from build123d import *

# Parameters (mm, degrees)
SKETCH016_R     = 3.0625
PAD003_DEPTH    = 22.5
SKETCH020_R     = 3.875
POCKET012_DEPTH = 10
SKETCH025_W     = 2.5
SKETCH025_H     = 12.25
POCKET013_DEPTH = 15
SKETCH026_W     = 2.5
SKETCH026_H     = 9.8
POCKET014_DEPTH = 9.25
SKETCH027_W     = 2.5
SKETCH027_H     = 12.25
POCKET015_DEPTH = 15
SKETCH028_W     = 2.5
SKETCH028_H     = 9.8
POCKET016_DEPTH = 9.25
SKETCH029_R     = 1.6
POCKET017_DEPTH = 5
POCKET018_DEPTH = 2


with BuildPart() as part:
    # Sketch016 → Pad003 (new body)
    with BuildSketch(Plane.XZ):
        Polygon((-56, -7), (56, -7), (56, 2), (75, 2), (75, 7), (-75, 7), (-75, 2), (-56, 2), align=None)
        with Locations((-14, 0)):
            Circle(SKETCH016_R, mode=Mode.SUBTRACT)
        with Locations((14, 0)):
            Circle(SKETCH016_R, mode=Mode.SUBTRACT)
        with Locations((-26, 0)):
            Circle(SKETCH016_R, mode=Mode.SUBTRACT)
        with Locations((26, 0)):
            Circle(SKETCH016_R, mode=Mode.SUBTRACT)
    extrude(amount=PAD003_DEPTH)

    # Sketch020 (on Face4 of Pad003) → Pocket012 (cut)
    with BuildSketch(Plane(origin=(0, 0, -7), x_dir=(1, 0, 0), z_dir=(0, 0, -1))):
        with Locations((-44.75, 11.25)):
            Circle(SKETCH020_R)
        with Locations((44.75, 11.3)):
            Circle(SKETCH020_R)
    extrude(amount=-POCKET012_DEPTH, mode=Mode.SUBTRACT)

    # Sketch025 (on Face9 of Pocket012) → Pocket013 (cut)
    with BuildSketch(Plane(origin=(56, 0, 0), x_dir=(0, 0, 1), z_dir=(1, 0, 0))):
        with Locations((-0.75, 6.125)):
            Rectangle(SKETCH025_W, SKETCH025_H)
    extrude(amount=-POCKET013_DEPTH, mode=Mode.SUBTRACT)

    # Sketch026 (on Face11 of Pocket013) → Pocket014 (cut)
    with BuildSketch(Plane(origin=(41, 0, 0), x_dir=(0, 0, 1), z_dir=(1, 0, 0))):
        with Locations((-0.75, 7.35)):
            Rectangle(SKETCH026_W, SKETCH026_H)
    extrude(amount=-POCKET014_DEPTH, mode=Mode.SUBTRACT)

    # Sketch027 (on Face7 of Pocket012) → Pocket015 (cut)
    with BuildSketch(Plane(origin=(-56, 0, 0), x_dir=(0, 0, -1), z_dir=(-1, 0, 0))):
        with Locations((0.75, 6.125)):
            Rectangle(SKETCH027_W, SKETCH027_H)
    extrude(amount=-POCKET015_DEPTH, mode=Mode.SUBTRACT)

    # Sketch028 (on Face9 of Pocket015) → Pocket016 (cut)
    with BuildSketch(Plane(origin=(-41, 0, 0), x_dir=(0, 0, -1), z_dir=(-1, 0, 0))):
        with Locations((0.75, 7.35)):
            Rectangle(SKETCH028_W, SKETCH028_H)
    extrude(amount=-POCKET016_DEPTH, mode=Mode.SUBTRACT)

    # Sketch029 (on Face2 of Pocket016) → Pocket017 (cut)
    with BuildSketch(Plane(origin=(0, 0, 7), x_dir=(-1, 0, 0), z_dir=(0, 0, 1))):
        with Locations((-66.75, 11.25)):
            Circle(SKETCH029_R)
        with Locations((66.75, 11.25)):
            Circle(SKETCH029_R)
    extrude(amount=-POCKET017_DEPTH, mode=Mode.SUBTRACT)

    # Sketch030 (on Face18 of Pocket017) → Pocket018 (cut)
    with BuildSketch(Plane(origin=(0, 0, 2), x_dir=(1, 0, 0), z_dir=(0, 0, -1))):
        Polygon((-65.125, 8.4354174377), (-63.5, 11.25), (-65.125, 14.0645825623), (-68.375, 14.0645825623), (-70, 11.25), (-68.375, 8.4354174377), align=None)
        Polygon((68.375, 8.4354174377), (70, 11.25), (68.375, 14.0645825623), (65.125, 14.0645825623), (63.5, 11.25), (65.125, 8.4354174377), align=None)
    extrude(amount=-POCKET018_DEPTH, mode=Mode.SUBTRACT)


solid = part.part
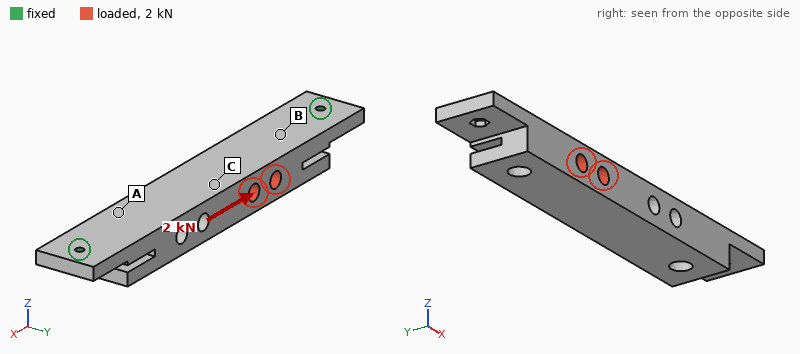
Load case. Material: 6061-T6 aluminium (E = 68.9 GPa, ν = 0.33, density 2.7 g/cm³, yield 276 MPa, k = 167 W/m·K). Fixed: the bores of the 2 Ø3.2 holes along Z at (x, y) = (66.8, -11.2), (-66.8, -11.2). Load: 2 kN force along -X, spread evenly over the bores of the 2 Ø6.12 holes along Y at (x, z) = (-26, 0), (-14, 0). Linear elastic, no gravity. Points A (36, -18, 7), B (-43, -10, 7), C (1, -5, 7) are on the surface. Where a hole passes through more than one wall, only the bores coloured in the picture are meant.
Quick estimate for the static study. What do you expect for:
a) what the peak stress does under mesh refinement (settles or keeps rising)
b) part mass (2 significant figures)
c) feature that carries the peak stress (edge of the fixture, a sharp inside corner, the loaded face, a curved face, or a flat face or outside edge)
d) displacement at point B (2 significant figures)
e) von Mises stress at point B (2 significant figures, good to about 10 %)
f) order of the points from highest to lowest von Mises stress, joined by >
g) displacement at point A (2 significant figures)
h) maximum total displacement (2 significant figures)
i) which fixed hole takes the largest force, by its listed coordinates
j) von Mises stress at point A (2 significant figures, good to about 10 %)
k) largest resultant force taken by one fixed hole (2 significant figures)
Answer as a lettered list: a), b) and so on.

a) keeps rising
b) 93 g
c) edge of the fixture
d) 6.5 µm
e) 9.3 MPa
f) B > A > C
g) 4.7 µm
h) 9.2 µm
i) (-66.8, -11.2)
j) 6.1 MPa
k) 1.1 kN
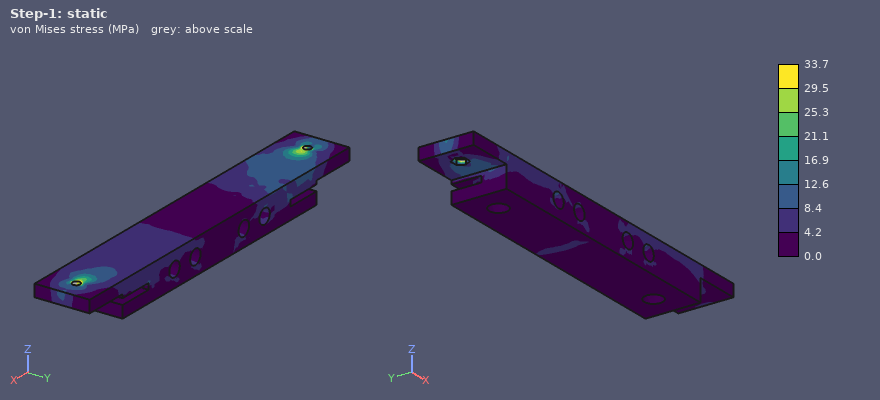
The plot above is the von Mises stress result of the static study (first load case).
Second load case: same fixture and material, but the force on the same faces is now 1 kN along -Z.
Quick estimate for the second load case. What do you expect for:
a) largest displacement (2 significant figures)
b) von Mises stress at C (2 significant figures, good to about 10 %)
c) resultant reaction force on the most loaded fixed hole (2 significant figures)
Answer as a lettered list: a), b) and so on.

a) 98 µm
b) 14 MPa
c) 1.4 kN
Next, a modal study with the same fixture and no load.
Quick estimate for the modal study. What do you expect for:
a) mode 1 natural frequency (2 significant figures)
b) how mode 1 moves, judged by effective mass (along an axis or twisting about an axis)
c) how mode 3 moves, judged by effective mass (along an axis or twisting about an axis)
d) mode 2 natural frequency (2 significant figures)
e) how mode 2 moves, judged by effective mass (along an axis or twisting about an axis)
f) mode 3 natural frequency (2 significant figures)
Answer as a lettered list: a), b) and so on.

a) 2100 Hz
b) along Y
c) along Y
d) 2200 Hz
e) along Z
f) 3700 Hz
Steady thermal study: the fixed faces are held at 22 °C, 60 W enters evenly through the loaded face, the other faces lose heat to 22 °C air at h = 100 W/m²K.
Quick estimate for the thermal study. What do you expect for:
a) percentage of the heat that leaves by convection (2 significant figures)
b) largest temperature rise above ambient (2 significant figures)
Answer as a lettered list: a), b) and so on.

a) 48 %
b) 41 K
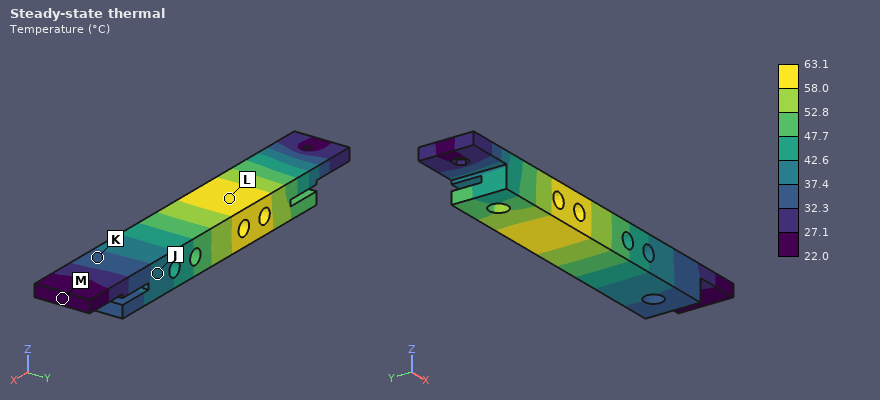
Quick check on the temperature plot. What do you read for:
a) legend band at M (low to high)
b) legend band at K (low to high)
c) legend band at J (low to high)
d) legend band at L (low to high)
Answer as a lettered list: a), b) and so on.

a) 22.0 to 27.1 °C
b) 32.3 to 37.4 °C
c) 37.4 to 42.6 °C
d) 58.0 to 63.1 °C
